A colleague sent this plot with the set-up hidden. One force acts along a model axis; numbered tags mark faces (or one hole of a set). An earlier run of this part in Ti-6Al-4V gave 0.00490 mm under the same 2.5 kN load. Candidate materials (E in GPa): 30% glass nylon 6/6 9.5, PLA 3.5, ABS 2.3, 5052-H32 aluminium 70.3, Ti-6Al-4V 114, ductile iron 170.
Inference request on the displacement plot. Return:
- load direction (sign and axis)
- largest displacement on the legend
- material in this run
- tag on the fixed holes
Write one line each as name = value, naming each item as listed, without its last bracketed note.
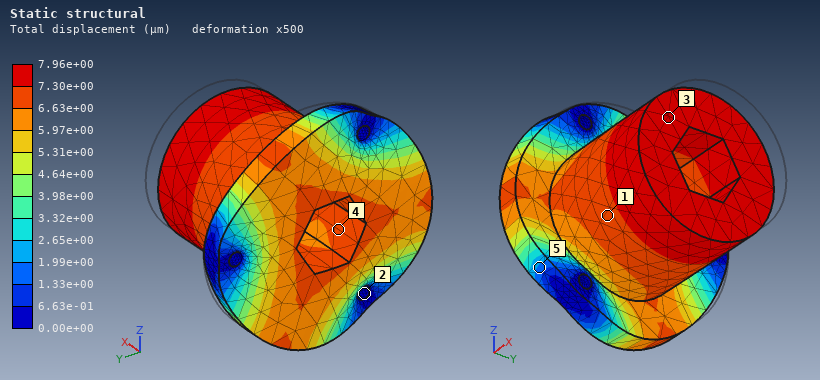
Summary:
load direction = -X
largest displacement on the legend = 7.96e+00 µm
material in this run = 5052-H32 aluminium
tag on the fixed holes = 2
